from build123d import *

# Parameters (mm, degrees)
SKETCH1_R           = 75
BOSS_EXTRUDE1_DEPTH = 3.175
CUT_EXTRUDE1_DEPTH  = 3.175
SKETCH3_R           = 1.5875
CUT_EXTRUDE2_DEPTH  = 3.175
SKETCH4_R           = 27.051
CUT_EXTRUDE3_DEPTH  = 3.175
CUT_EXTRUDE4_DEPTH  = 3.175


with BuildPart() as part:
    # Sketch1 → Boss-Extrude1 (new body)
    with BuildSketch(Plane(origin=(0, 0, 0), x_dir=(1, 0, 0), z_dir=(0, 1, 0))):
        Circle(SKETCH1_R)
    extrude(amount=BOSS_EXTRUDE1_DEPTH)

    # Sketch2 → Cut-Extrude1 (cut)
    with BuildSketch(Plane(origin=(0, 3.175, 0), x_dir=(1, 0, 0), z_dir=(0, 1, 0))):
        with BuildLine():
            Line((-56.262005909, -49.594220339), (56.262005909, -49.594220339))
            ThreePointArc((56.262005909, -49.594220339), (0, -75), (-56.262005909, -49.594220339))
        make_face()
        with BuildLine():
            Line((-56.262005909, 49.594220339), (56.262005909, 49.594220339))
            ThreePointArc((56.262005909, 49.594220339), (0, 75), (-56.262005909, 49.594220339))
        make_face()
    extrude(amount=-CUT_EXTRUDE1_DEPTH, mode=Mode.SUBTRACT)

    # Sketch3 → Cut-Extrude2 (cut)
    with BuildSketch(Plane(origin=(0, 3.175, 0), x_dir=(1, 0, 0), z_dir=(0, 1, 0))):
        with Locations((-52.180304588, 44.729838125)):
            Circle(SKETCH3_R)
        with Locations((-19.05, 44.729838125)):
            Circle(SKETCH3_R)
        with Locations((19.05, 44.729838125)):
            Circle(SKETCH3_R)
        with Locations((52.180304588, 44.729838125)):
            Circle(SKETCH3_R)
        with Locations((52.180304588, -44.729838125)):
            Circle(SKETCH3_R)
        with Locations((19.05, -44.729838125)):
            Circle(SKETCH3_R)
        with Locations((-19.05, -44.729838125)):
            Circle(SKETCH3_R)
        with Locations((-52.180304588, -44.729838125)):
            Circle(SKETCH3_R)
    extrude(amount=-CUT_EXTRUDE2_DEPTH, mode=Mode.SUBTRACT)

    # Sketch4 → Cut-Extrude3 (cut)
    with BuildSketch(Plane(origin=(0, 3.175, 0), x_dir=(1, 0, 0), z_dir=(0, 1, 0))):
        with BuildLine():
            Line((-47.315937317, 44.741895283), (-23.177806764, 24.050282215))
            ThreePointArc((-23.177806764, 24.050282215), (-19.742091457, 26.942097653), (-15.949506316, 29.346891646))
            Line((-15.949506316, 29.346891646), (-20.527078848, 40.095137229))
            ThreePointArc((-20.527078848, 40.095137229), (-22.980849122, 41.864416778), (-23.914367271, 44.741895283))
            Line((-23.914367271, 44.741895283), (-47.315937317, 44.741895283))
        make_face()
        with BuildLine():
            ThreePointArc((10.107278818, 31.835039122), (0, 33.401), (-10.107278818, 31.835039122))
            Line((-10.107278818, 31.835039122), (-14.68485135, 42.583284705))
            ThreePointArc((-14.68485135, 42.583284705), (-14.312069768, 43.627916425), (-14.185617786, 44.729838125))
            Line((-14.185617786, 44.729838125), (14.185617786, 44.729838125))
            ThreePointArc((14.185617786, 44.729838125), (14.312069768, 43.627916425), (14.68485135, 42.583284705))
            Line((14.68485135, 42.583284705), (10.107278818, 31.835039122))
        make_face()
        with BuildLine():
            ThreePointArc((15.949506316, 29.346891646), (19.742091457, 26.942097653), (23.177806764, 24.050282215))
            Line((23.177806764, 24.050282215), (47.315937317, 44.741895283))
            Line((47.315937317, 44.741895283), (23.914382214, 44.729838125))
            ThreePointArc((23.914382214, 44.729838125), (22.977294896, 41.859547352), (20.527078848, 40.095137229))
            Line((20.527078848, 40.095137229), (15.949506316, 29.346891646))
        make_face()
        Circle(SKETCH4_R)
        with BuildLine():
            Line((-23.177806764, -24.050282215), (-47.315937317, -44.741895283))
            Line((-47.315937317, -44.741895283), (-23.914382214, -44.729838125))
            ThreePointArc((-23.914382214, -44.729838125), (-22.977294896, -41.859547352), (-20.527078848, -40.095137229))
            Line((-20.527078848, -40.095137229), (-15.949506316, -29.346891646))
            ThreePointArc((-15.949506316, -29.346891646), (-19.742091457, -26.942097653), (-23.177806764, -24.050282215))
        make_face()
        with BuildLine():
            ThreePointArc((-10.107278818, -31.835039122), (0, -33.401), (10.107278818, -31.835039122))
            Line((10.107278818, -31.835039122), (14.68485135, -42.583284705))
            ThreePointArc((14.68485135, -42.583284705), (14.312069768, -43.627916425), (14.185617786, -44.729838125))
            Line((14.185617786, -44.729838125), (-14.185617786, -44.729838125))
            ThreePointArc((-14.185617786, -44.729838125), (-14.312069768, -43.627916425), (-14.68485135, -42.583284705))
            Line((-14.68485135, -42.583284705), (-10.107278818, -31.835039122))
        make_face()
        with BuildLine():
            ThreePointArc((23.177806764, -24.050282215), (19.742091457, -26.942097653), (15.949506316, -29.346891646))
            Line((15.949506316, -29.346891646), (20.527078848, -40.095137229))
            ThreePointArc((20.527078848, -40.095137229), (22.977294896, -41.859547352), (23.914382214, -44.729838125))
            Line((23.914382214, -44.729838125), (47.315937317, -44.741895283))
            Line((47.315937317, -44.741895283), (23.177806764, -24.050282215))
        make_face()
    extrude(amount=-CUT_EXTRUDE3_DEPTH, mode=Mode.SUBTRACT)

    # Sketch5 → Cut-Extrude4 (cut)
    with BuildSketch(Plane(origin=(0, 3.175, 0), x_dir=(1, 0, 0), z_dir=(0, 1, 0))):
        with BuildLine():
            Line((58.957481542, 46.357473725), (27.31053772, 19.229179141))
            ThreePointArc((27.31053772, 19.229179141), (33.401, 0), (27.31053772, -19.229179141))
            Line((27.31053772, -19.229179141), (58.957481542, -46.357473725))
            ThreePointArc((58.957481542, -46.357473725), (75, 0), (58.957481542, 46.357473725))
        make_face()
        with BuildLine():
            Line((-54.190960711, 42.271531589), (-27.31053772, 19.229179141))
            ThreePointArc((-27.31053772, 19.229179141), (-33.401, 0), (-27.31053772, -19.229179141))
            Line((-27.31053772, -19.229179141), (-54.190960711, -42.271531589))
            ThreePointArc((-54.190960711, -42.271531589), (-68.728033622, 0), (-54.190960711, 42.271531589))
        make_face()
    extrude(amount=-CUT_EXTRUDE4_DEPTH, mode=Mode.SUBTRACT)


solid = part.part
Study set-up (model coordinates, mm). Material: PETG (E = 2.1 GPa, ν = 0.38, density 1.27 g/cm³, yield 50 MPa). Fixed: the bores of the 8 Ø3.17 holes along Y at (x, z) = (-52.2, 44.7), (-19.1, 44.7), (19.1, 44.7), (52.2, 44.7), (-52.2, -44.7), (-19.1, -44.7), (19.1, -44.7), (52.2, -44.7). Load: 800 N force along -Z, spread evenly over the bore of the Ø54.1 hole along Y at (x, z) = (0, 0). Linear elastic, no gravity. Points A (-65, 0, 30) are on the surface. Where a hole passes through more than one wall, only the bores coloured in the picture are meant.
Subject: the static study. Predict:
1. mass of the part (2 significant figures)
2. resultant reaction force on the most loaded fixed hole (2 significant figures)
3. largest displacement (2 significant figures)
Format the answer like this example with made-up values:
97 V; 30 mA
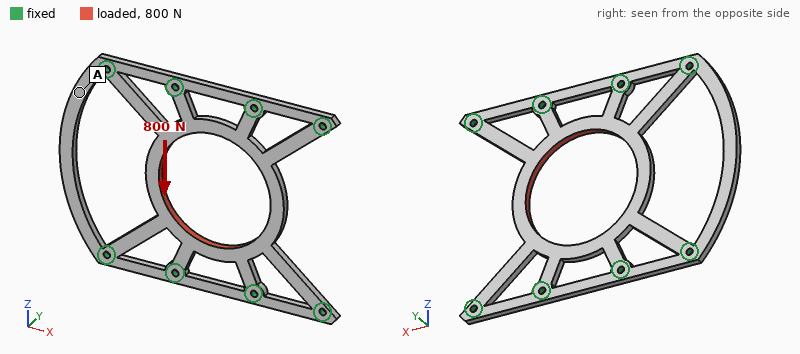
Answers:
17 g; 160 N; 0.17 mm
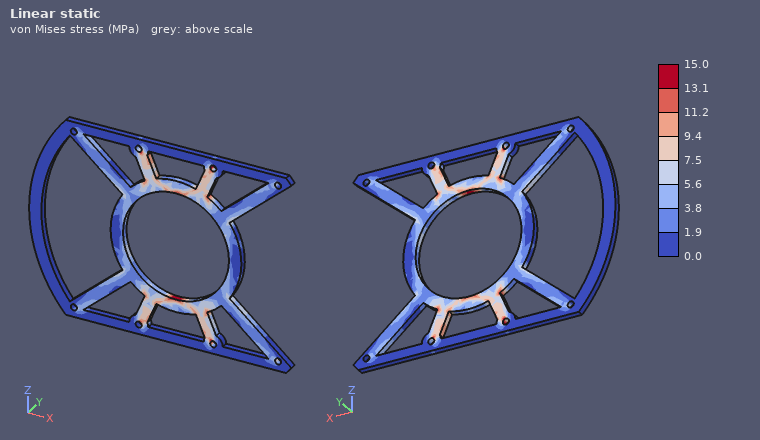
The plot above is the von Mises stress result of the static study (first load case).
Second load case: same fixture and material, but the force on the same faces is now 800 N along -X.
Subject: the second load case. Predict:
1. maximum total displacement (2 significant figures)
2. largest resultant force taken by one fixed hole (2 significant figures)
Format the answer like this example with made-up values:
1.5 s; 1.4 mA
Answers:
0.67 mm; 150 N
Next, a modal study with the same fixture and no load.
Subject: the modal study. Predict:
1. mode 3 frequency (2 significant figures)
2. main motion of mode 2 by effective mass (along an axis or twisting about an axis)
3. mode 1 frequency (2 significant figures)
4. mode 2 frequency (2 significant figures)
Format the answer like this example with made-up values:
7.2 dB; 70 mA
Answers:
590 Hz; along Y; 390 Hz; 520 Hz
